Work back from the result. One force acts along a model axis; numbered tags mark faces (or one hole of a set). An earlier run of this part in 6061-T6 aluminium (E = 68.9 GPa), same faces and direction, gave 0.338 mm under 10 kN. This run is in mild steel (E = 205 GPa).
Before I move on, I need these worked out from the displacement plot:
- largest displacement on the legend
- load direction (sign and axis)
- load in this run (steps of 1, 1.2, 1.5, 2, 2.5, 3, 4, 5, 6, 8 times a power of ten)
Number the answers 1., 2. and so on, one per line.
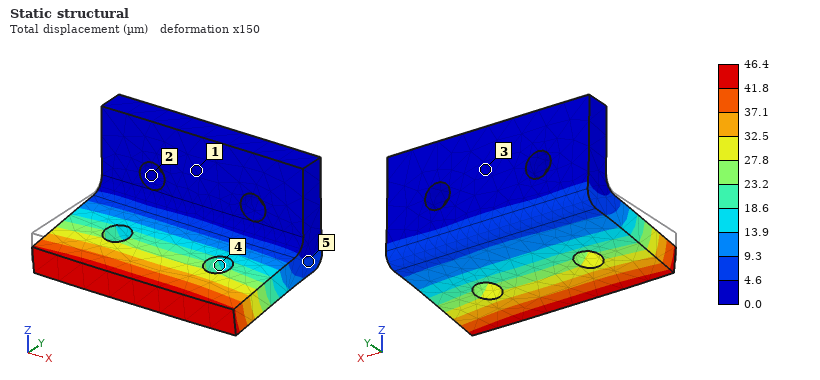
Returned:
1. 46.4 µm
2. -Z
3. 4 kN
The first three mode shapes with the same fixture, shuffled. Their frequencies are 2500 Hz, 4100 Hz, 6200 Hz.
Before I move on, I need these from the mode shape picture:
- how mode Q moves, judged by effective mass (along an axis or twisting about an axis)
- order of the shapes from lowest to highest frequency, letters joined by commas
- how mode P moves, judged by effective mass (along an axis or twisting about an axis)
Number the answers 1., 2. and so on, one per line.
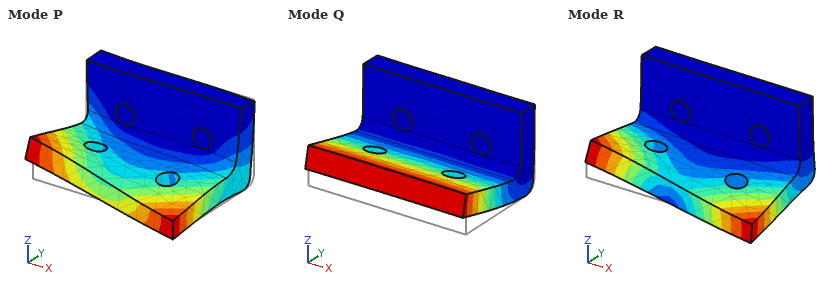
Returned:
1. along Z
2. Q, R, P
3. along X
